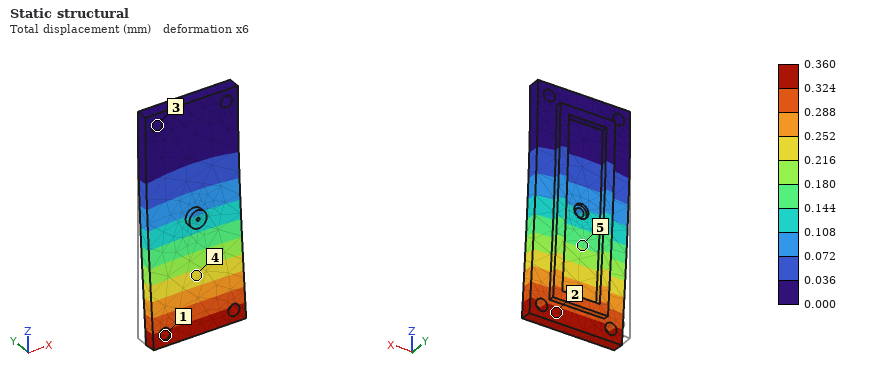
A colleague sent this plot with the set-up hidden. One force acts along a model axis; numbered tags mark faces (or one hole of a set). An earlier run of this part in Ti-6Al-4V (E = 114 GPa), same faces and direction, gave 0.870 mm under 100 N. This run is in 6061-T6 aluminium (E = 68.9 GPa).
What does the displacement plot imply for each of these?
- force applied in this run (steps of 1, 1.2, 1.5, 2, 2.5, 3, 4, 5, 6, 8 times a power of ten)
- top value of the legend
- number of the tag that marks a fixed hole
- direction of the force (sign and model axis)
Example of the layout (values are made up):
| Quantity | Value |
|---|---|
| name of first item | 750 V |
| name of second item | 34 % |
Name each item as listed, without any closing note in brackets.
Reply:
| Quantity | Value |
|---|---|
| force applied in this run | 25 N |
| top value of the legend | 0.360 mm |
| number of the tag that marks a fixed hole | 3 |
| direction of the force | -Y |
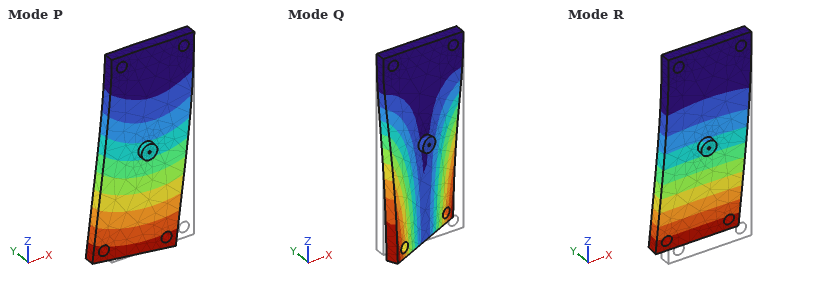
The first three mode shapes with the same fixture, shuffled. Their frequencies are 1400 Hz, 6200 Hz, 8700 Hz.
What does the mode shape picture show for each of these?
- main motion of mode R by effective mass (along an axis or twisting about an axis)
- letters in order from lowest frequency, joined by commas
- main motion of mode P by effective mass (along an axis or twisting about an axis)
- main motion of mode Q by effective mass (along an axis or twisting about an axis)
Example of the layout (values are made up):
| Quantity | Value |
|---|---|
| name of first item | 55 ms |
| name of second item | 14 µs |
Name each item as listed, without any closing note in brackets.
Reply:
| Quantity | Value |
|---|---|
| main motion of mode R by effective mass | along Y |
| letters in order from lowest frequency, joined by commas | R, Q, P |
| main motion of mode P by effective mass | along X |
| main motion of mode Q by effective mass | twisting about Z |
